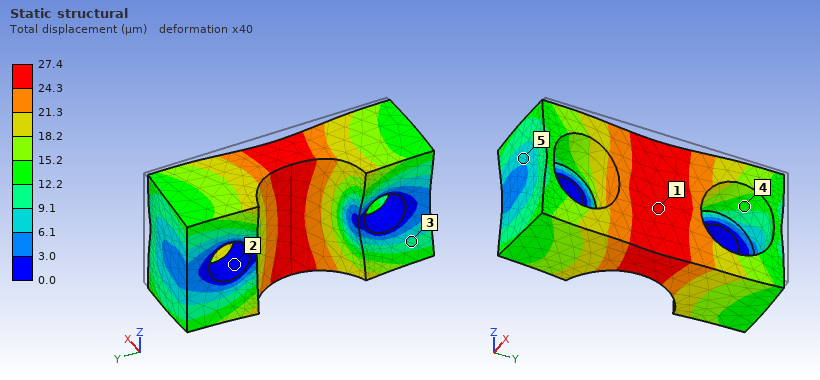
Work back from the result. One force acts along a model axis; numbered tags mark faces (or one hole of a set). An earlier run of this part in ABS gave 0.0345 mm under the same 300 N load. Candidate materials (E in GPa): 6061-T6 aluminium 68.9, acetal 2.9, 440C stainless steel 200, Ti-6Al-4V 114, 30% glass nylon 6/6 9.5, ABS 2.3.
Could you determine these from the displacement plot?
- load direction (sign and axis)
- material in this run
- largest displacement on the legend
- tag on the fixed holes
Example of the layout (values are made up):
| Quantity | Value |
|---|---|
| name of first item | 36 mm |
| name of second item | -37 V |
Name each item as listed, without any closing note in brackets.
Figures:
| Quantity | Value |
|---|---|
| load direction | -X |
| material in this run | acetal |
| largest displacement on the legend | 27.4 µm |
| tag on the fixed holes | 2 |
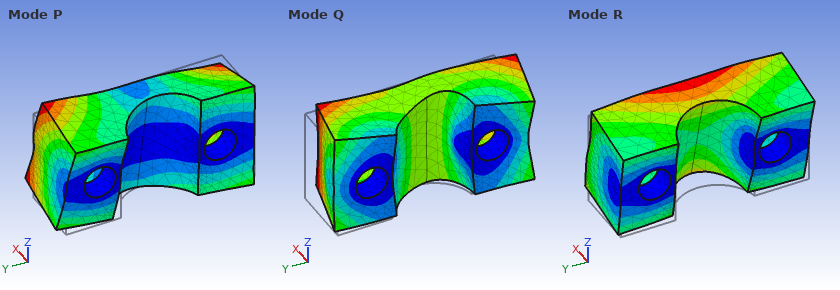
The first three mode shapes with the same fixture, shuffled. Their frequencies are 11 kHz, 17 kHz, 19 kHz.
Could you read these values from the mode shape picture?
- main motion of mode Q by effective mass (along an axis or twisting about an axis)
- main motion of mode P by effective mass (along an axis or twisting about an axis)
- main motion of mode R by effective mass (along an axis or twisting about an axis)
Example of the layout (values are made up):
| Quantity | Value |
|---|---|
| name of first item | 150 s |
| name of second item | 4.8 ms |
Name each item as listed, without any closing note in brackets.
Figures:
| Quantity | Value |
|---|---|
| main motion of mode Q by effective mass | along Y |
| main motion of mode P by effective mass | twisting about X |
| main motion of mode R by effective mass | along Z |
